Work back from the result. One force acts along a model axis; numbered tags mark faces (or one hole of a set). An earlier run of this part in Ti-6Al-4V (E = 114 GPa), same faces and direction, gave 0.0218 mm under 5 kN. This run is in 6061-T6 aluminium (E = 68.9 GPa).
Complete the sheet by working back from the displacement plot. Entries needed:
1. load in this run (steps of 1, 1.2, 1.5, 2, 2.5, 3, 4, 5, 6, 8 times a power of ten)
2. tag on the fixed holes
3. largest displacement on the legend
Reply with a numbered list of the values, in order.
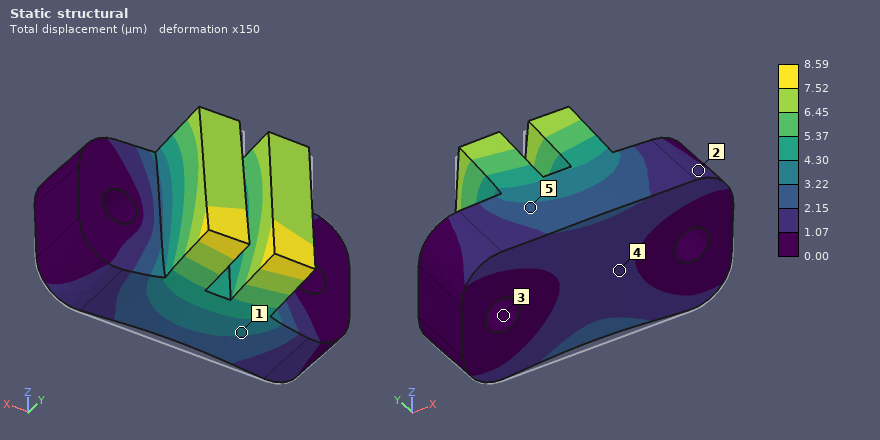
1. 1.2 kN
2. 3
3. 8.59 µm
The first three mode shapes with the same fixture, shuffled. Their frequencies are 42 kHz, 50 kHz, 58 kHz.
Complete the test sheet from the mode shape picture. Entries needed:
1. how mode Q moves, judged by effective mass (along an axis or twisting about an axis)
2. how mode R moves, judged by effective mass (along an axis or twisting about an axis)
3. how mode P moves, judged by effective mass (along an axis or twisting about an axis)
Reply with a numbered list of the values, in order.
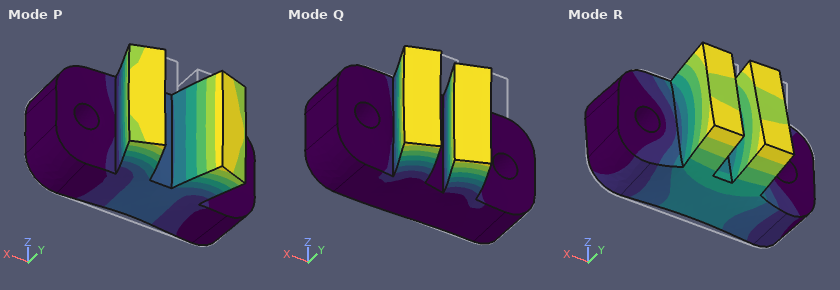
1. along X
2. along Z
3. along Y
